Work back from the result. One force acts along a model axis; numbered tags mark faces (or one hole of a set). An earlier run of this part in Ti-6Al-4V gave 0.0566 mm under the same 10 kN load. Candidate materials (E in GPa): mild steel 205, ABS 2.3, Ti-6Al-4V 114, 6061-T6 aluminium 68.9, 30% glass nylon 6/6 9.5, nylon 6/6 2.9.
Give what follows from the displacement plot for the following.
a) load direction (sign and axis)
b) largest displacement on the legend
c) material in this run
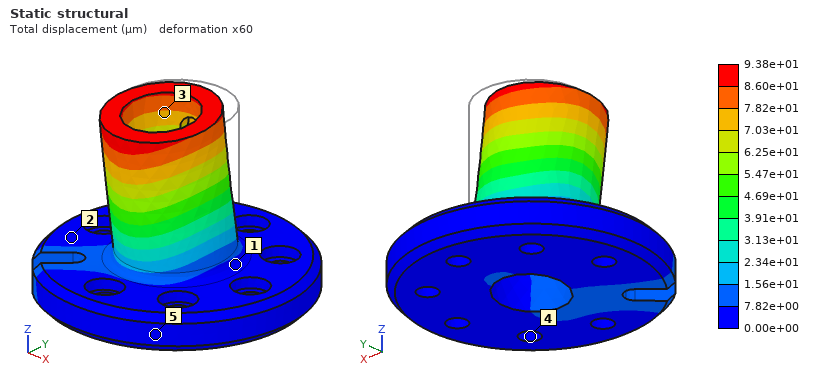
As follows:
-Y
9.38e+01 µm
6061-T6 aluminium
